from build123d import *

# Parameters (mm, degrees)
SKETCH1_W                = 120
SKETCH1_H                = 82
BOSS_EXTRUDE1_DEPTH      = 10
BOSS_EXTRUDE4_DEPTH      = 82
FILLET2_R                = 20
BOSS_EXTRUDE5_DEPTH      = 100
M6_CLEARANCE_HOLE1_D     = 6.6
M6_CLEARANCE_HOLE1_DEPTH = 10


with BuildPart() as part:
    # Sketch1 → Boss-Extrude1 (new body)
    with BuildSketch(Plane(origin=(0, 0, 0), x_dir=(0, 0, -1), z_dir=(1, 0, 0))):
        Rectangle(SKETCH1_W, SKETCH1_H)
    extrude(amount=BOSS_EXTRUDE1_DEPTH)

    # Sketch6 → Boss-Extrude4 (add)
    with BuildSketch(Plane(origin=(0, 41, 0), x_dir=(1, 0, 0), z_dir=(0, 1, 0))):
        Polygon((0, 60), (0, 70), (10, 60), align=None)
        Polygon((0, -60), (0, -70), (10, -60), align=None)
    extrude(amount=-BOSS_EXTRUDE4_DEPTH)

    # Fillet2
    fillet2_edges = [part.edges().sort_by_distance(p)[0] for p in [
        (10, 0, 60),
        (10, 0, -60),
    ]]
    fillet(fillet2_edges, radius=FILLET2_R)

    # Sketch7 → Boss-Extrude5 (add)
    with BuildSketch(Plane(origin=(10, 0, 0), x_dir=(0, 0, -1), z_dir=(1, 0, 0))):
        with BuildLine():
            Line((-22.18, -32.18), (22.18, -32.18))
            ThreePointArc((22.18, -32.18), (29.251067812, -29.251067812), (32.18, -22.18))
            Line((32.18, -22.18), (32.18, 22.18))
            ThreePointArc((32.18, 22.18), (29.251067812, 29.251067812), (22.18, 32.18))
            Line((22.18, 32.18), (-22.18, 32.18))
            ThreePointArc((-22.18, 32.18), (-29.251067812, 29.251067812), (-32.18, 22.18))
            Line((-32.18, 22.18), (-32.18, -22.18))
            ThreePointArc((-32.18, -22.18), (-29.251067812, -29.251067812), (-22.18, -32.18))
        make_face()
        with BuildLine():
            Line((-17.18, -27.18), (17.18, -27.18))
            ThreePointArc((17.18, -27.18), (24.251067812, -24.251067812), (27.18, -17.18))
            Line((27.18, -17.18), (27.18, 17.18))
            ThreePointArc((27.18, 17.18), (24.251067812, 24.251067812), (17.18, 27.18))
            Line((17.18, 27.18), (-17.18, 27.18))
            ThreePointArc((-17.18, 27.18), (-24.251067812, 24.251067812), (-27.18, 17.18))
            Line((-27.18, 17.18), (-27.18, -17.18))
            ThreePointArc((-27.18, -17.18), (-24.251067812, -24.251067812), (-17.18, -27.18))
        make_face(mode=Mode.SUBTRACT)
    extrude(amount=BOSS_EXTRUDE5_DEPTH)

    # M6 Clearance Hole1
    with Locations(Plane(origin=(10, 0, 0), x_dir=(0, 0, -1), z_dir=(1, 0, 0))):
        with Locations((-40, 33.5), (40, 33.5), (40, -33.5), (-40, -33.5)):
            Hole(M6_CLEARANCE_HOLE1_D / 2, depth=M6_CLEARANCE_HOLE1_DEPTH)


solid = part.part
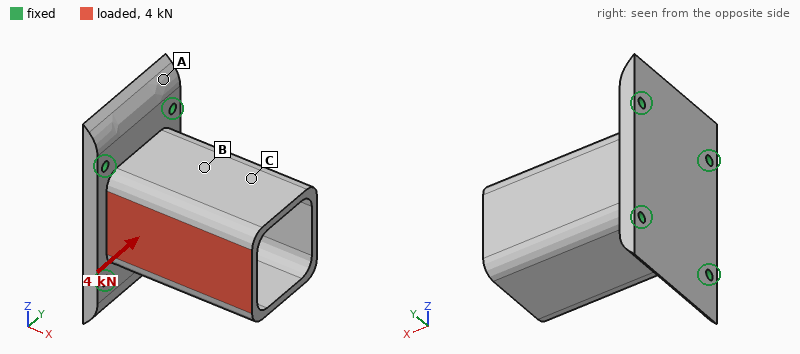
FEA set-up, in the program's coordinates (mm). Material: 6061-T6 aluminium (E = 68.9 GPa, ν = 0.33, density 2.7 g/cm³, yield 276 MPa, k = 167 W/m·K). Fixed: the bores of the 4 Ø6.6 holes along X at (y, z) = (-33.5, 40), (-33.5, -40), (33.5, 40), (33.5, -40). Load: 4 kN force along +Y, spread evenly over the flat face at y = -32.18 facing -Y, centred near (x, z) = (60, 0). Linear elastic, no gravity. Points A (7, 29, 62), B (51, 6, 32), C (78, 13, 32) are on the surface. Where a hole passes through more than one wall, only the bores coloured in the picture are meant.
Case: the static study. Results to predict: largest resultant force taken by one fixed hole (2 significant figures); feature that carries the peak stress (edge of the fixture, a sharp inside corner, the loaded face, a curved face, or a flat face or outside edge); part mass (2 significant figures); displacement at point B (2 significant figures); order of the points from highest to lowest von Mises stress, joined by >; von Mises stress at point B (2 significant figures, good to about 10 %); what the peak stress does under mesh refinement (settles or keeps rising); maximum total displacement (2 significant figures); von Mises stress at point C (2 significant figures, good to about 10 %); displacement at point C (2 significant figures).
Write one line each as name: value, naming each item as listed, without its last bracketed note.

largest resultant force taken by one fixed hole: 2.1 kN
feature that carries the peak stress: edge of the fixture
part mass: 600 g
displacement at point B: 0.035 mm
order of the points from highest to lowest von Mises stress, joined by >: B > C > A
von Mises stress at point B: 12 MPa
what the peak stress does under mesh refinement: keeps rising
maximum total displacement: 0.14 mm
von Mises stress at point C: 6.7 MPa
displacement at point C: 0.052 mm
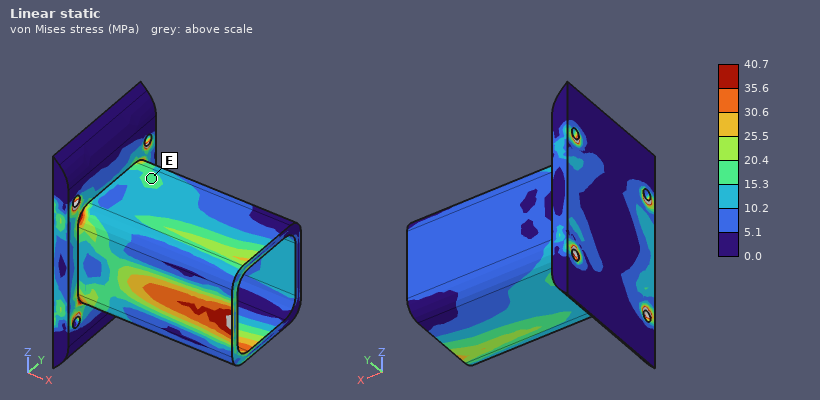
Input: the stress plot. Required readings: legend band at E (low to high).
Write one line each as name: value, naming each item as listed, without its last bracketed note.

legend band at E: 15.3 to 20.4 MPa
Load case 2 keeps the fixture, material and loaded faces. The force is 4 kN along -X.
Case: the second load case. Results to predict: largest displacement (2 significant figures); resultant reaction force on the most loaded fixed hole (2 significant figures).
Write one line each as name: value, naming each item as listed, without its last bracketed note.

largest displacement: 51 µm
resultant reaction force on the most loaded fixed hole: 2.1 kN
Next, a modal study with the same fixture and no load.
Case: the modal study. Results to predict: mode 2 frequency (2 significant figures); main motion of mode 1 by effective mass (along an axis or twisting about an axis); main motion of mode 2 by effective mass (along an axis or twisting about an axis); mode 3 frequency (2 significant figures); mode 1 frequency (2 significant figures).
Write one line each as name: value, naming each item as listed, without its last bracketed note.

mode 2 frequency: 2800 Hz
main motion of mode 1 by effective mass: along Y
main motion of mode 2 by effective mass: along Z
mode 3 frequency: 3500 Hz
mode 1 frequency: 2500 Hz
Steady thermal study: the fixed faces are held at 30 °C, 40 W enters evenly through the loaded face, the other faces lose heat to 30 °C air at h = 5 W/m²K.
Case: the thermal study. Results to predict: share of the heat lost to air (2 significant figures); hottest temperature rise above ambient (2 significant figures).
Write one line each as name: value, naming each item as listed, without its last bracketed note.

share of the heat lost to air: 5.5 %
hottest temperature rise above ambient: 18 K
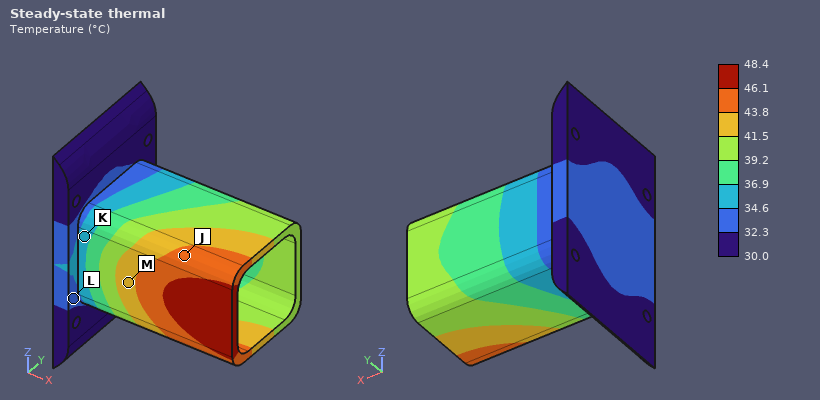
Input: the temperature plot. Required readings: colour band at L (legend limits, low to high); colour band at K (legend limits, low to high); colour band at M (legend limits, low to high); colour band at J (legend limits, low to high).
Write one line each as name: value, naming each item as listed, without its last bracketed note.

colour band at L: 32.3 to 34.6 °C
colour band at K: 34.6 to 36.9 °C
colour band at M: 41.5 to 43.8 °C
colour band at J: 43.8 to 46.1 °C
